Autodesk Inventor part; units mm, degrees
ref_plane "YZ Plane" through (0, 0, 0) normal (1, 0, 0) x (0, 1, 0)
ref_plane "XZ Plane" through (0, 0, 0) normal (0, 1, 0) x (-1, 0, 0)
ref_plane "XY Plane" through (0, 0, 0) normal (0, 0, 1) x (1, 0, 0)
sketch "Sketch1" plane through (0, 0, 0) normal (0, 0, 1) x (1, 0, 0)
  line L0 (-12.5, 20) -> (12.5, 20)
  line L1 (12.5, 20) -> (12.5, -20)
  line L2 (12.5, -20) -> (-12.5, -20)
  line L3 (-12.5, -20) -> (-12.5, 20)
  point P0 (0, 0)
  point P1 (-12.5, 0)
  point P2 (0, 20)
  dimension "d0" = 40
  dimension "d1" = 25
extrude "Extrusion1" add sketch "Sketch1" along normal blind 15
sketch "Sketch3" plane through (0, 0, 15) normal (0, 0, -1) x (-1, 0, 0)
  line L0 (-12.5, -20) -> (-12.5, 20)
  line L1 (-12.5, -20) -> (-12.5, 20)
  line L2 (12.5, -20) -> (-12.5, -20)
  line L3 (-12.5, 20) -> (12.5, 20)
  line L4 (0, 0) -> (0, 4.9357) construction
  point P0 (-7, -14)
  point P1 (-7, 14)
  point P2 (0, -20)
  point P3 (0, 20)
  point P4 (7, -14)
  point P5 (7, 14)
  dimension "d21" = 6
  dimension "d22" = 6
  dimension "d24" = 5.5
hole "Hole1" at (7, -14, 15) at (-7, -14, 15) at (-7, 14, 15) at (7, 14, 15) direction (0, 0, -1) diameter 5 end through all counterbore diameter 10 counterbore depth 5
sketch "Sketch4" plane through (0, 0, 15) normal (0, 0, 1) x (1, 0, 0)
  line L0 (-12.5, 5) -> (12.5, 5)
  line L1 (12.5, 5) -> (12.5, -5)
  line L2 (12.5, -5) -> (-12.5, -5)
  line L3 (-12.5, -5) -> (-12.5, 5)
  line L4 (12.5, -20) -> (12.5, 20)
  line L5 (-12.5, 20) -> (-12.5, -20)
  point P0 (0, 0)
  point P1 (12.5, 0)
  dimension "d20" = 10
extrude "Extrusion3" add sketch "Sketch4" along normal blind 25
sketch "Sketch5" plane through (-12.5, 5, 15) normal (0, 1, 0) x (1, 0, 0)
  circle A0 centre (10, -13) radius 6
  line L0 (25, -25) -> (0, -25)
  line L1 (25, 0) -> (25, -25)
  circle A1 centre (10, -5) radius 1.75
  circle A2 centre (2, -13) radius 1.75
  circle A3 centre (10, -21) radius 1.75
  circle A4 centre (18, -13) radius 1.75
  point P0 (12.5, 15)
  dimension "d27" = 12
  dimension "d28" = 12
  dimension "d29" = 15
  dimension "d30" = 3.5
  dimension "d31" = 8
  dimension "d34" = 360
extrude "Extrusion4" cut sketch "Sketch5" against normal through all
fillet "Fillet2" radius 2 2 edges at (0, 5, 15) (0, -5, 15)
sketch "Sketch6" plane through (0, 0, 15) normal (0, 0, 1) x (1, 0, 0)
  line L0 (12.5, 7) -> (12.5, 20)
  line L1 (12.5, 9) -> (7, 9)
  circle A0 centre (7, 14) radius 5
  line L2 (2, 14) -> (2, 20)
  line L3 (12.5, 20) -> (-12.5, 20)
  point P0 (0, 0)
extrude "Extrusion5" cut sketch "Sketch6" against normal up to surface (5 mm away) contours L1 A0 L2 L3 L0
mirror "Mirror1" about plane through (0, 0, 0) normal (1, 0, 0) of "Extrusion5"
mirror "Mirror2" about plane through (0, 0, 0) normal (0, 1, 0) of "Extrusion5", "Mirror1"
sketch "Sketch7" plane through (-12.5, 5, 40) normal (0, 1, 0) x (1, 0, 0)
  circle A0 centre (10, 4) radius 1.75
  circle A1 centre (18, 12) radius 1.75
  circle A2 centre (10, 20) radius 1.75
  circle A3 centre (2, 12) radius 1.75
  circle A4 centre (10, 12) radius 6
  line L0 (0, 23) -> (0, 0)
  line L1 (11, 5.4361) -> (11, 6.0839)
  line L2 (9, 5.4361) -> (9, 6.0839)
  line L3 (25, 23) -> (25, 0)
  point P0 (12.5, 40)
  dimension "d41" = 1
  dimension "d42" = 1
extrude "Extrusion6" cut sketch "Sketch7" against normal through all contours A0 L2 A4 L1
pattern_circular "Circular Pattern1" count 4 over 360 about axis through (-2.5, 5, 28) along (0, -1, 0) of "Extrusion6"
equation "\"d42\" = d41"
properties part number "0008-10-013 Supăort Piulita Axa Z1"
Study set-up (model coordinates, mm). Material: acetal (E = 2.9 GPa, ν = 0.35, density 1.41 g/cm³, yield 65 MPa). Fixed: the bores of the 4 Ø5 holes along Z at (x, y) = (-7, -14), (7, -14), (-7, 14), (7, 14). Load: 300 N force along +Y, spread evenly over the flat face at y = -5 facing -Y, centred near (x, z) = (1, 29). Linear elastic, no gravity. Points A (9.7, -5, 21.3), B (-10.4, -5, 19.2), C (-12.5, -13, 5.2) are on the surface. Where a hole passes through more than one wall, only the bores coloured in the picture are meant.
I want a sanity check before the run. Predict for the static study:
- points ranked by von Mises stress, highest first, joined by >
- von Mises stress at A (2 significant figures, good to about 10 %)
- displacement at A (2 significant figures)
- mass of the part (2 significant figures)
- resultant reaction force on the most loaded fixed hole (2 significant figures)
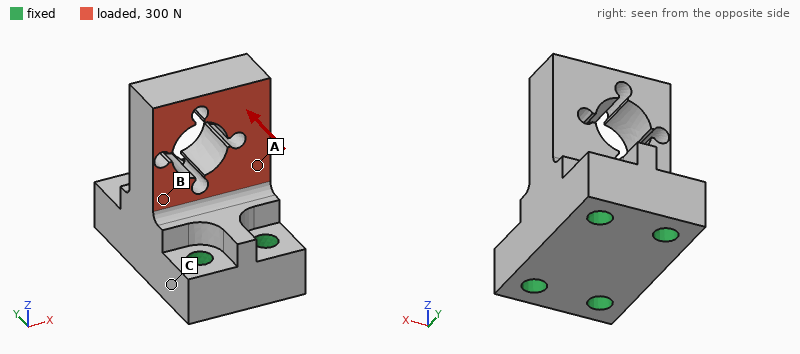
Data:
A > B > C
12 MPa
0.066 mm
24 g
170 N
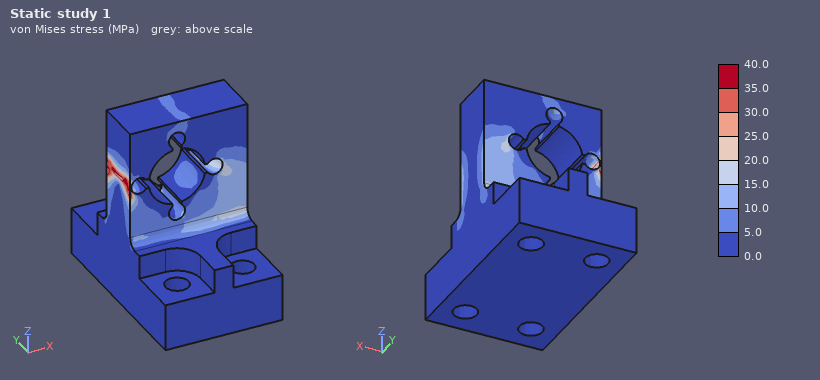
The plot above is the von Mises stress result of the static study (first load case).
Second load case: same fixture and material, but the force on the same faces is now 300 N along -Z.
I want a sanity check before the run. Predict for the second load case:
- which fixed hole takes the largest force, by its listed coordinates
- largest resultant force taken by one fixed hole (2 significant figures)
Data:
(7, -14)
120 N
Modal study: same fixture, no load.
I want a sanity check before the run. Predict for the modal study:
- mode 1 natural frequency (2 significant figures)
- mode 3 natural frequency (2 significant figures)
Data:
2200 Hz
4200 Hz
